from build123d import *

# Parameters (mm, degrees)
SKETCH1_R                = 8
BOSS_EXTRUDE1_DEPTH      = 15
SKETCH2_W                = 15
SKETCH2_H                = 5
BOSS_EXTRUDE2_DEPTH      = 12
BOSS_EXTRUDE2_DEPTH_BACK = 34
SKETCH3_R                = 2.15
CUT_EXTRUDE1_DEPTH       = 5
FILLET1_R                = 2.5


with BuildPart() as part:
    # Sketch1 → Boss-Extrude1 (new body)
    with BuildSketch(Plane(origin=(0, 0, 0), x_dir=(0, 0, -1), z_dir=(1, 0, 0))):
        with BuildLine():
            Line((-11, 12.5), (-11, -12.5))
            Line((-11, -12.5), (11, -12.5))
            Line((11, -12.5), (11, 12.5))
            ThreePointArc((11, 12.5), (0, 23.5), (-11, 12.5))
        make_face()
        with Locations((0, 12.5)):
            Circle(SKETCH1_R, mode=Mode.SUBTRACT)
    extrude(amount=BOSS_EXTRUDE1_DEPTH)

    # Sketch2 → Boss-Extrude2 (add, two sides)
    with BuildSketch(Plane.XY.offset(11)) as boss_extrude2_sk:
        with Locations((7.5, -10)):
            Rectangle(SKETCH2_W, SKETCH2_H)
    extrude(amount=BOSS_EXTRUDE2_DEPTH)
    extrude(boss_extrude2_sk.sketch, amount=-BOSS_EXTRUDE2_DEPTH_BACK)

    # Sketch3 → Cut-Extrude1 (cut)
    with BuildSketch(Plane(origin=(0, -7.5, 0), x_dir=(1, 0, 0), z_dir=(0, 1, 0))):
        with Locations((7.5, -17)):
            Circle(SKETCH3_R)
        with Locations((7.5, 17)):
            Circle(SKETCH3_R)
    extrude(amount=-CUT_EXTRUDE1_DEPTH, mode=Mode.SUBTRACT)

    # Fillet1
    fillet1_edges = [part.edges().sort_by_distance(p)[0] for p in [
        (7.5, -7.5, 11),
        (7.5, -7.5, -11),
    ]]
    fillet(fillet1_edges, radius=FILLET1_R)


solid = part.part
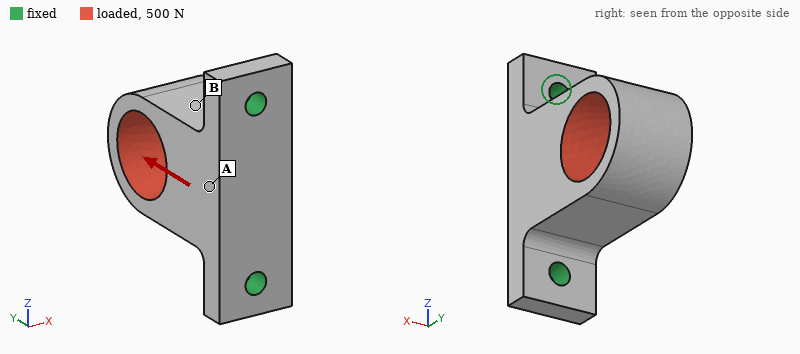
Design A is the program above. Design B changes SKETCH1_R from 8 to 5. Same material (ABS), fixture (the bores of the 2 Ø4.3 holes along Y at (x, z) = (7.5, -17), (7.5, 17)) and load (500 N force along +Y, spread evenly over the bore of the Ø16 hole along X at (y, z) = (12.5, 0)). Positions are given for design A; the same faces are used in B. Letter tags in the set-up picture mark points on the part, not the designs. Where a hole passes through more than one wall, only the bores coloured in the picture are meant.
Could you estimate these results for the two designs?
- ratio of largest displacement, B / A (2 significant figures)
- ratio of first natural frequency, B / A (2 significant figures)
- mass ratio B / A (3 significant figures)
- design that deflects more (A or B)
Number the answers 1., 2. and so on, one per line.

1. 0.62
2. 0.82
3. 1.19
4. A
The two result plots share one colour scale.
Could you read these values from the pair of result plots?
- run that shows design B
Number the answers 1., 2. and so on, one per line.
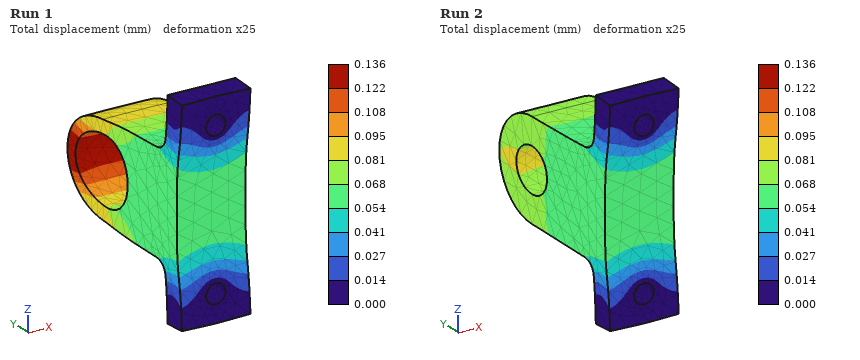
1. Run 2
